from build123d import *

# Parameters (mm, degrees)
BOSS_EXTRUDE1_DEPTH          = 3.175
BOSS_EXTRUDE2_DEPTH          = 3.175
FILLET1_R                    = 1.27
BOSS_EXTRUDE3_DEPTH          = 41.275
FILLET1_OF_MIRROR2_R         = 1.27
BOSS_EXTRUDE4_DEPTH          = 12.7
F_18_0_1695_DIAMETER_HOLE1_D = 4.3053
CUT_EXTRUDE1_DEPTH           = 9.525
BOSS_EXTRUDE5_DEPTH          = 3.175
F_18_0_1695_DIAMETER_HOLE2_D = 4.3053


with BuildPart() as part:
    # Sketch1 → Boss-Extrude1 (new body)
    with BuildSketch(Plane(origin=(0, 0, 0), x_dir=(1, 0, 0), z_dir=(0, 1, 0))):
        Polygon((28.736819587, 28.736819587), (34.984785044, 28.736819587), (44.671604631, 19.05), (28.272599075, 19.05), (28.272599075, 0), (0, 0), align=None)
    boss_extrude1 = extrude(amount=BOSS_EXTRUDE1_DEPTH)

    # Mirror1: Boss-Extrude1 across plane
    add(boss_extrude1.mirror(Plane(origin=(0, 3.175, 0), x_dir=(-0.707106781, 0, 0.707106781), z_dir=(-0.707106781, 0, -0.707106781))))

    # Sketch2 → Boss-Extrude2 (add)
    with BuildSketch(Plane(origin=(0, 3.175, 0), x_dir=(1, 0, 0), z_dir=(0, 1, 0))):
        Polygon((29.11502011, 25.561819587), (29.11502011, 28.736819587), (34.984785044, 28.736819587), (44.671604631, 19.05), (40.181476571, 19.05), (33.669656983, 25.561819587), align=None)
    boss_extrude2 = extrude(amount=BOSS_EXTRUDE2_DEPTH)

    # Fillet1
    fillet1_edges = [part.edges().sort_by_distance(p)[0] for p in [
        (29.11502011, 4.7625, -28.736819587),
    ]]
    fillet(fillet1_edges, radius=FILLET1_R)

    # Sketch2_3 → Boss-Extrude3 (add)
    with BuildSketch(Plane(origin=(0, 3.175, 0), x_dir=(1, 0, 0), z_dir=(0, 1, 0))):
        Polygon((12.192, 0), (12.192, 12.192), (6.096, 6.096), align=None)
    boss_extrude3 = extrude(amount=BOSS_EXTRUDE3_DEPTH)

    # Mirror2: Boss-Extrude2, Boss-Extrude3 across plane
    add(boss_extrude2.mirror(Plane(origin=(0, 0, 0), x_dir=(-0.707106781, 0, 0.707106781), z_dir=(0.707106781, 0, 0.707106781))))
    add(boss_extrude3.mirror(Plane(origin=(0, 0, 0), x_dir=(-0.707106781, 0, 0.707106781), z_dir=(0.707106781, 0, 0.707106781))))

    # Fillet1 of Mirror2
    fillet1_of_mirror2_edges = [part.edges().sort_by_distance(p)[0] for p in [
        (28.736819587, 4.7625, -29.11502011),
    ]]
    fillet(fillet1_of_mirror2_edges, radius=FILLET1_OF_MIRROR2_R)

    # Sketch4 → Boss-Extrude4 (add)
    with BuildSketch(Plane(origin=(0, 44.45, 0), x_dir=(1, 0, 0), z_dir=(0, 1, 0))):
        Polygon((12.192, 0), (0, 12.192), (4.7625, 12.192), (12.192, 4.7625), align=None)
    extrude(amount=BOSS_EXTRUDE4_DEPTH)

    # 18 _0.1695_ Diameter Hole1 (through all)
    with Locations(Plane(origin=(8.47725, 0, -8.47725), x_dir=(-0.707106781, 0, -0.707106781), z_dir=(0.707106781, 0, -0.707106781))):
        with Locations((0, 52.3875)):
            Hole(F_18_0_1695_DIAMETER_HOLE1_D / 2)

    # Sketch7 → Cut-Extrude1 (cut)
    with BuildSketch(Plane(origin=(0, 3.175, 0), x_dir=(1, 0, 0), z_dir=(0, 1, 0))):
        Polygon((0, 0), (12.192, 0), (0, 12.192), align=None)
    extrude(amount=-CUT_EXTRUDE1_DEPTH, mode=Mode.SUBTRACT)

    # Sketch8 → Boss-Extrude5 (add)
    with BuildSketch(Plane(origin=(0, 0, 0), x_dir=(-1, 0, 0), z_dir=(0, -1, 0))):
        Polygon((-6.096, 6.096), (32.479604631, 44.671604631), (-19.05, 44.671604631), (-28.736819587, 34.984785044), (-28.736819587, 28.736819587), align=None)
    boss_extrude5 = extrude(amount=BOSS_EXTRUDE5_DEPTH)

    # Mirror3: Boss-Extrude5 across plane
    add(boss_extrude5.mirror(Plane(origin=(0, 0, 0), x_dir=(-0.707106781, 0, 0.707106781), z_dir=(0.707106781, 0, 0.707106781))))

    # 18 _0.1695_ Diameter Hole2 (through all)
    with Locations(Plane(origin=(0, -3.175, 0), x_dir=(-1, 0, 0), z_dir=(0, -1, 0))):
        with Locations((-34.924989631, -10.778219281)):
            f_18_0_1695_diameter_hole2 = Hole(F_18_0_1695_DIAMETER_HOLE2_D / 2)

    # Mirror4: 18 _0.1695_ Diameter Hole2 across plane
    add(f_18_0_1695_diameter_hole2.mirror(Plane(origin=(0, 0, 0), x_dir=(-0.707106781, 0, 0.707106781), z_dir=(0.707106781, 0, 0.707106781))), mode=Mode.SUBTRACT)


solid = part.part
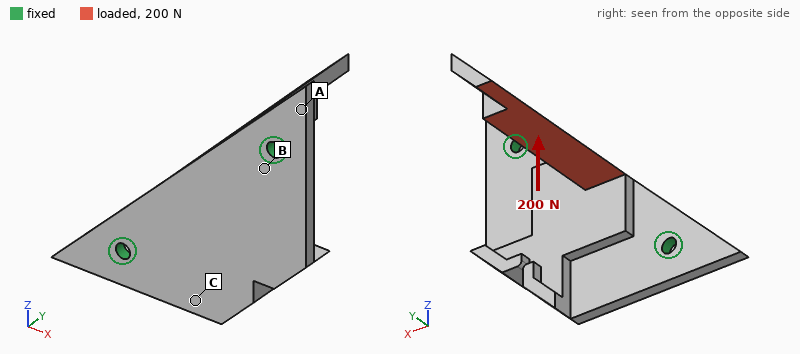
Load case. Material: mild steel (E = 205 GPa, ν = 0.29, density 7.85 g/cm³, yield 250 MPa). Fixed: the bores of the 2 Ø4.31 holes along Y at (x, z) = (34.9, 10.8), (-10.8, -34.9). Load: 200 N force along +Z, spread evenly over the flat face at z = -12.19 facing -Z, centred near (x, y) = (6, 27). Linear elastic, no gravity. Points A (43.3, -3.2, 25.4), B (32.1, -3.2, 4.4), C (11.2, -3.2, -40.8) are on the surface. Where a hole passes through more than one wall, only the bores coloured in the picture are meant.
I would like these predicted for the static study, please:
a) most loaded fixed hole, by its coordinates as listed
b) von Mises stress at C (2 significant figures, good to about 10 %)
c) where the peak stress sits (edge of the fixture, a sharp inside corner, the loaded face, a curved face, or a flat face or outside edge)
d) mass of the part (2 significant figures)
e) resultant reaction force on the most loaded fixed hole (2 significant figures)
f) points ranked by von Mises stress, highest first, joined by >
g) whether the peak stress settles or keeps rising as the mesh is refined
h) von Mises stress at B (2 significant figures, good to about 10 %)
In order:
(34.9, 10.8)
18 MPa
edge of the fixture
120 g
170 N
B > C > A
keeps rising
43 MPa
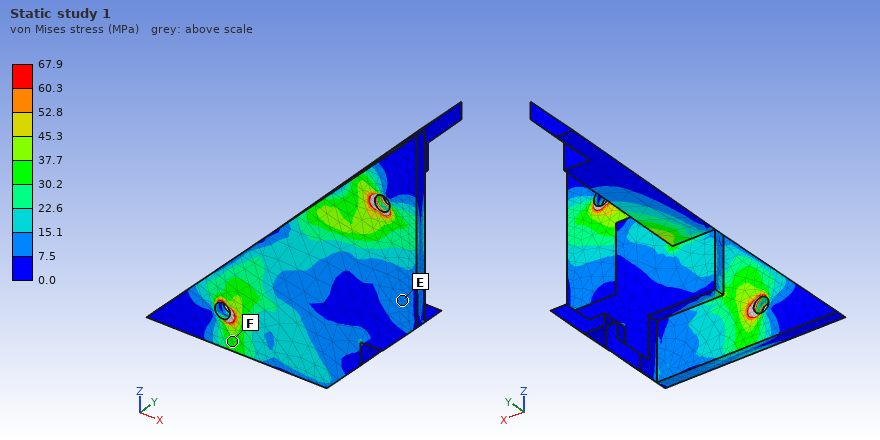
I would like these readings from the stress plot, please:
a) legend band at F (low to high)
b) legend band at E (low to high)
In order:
30.2 to 37.7 MPa
7.5 to 15.1 MPa
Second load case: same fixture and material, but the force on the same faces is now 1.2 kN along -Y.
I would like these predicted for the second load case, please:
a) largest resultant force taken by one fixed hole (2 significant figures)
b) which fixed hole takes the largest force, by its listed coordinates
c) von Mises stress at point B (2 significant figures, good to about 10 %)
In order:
1.1 kN
(-10.8, -34.9)
100 MPa
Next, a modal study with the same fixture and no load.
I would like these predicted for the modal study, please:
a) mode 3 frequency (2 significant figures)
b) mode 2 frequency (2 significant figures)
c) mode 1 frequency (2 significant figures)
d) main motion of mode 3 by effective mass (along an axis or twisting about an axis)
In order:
2800 Hz
2300 Hz
1100 Hz
along Y
